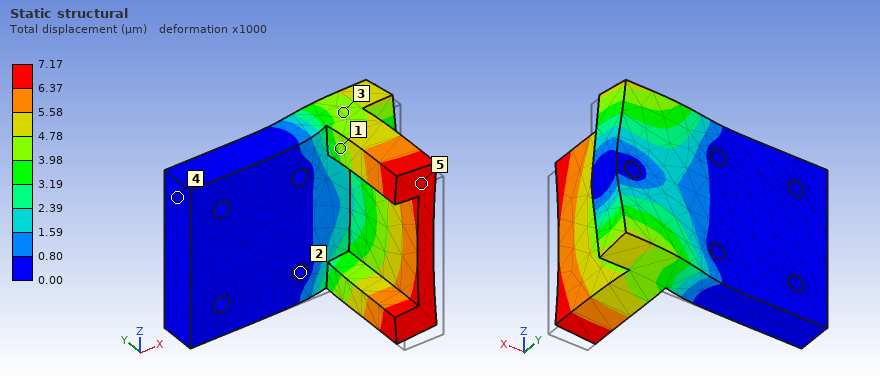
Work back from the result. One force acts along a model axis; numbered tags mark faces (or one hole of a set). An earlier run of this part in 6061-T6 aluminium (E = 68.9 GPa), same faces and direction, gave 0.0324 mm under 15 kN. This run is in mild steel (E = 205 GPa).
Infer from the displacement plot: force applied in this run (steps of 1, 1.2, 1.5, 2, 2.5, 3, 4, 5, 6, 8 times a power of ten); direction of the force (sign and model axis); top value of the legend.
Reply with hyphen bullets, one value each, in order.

- 10 kN
- +Y
- 7.17 µm
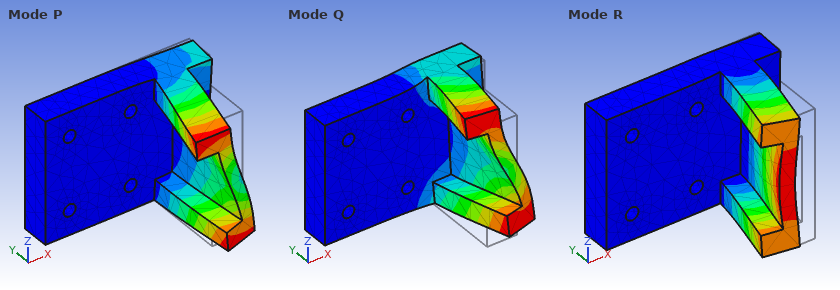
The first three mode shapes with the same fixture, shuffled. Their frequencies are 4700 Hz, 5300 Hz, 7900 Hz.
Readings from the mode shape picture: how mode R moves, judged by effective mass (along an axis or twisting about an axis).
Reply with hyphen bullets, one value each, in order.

- along X
